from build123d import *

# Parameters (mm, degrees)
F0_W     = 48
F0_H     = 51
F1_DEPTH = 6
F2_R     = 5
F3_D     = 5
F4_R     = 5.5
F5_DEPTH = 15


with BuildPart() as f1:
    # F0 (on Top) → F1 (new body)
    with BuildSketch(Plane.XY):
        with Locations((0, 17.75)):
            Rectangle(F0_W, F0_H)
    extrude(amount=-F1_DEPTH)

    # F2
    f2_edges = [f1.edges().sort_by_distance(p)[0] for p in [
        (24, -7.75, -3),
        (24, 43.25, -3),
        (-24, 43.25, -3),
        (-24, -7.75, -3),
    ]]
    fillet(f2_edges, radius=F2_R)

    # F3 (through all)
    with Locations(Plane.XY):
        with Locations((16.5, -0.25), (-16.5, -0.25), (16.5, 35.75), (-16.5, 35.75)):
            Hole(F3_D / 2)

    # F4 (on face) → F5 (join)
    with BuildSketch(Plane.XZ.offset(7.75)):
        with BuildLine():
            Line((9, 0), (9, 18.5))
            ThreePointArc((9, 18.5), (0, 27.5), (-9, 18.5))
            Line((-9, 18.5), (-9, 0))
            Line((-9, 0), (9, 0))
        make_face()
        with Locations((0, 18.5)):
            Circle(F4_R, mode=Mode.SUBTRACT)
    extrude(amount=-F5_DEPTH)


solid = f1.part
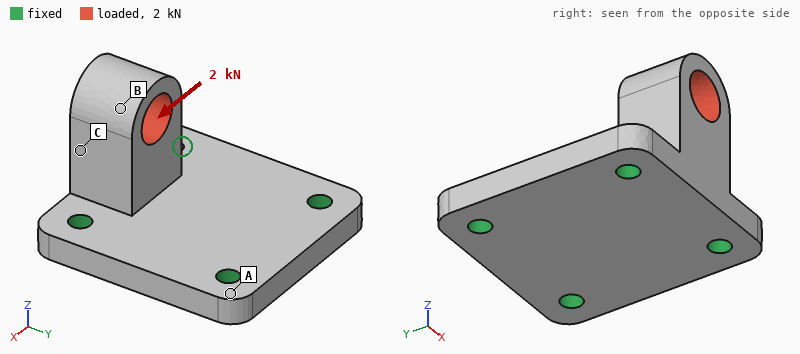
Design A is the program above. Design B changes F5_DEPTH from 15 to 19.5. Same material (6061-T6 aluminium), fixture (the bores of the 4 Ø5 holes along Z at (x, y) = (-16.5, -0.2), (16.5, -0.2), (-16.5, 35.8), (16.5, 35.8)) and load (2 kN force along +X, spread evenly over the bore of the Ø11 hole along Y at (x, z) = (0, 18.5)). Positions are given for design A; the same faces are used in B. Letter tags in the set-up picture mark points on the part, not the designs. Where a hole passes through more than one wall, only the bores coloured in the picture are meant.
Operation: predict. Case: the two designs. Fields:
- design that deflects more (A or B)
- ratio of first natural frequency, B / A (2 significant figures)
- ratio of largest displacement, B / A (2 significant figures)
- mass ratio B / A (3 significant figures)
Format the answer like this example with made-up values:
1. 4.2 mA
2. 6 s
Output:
1. A
2. 1.0
3. 0.82
4. 1.08
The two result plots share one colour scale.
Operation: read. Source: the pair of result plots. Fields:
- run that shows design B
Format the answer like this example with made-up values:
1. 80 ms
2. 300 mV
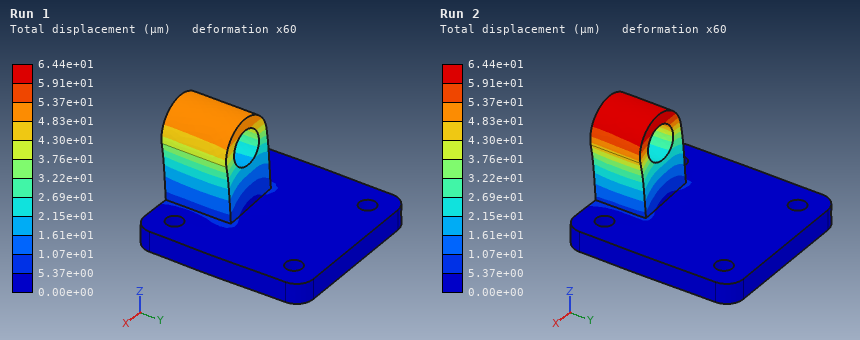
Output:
1. Run 1
